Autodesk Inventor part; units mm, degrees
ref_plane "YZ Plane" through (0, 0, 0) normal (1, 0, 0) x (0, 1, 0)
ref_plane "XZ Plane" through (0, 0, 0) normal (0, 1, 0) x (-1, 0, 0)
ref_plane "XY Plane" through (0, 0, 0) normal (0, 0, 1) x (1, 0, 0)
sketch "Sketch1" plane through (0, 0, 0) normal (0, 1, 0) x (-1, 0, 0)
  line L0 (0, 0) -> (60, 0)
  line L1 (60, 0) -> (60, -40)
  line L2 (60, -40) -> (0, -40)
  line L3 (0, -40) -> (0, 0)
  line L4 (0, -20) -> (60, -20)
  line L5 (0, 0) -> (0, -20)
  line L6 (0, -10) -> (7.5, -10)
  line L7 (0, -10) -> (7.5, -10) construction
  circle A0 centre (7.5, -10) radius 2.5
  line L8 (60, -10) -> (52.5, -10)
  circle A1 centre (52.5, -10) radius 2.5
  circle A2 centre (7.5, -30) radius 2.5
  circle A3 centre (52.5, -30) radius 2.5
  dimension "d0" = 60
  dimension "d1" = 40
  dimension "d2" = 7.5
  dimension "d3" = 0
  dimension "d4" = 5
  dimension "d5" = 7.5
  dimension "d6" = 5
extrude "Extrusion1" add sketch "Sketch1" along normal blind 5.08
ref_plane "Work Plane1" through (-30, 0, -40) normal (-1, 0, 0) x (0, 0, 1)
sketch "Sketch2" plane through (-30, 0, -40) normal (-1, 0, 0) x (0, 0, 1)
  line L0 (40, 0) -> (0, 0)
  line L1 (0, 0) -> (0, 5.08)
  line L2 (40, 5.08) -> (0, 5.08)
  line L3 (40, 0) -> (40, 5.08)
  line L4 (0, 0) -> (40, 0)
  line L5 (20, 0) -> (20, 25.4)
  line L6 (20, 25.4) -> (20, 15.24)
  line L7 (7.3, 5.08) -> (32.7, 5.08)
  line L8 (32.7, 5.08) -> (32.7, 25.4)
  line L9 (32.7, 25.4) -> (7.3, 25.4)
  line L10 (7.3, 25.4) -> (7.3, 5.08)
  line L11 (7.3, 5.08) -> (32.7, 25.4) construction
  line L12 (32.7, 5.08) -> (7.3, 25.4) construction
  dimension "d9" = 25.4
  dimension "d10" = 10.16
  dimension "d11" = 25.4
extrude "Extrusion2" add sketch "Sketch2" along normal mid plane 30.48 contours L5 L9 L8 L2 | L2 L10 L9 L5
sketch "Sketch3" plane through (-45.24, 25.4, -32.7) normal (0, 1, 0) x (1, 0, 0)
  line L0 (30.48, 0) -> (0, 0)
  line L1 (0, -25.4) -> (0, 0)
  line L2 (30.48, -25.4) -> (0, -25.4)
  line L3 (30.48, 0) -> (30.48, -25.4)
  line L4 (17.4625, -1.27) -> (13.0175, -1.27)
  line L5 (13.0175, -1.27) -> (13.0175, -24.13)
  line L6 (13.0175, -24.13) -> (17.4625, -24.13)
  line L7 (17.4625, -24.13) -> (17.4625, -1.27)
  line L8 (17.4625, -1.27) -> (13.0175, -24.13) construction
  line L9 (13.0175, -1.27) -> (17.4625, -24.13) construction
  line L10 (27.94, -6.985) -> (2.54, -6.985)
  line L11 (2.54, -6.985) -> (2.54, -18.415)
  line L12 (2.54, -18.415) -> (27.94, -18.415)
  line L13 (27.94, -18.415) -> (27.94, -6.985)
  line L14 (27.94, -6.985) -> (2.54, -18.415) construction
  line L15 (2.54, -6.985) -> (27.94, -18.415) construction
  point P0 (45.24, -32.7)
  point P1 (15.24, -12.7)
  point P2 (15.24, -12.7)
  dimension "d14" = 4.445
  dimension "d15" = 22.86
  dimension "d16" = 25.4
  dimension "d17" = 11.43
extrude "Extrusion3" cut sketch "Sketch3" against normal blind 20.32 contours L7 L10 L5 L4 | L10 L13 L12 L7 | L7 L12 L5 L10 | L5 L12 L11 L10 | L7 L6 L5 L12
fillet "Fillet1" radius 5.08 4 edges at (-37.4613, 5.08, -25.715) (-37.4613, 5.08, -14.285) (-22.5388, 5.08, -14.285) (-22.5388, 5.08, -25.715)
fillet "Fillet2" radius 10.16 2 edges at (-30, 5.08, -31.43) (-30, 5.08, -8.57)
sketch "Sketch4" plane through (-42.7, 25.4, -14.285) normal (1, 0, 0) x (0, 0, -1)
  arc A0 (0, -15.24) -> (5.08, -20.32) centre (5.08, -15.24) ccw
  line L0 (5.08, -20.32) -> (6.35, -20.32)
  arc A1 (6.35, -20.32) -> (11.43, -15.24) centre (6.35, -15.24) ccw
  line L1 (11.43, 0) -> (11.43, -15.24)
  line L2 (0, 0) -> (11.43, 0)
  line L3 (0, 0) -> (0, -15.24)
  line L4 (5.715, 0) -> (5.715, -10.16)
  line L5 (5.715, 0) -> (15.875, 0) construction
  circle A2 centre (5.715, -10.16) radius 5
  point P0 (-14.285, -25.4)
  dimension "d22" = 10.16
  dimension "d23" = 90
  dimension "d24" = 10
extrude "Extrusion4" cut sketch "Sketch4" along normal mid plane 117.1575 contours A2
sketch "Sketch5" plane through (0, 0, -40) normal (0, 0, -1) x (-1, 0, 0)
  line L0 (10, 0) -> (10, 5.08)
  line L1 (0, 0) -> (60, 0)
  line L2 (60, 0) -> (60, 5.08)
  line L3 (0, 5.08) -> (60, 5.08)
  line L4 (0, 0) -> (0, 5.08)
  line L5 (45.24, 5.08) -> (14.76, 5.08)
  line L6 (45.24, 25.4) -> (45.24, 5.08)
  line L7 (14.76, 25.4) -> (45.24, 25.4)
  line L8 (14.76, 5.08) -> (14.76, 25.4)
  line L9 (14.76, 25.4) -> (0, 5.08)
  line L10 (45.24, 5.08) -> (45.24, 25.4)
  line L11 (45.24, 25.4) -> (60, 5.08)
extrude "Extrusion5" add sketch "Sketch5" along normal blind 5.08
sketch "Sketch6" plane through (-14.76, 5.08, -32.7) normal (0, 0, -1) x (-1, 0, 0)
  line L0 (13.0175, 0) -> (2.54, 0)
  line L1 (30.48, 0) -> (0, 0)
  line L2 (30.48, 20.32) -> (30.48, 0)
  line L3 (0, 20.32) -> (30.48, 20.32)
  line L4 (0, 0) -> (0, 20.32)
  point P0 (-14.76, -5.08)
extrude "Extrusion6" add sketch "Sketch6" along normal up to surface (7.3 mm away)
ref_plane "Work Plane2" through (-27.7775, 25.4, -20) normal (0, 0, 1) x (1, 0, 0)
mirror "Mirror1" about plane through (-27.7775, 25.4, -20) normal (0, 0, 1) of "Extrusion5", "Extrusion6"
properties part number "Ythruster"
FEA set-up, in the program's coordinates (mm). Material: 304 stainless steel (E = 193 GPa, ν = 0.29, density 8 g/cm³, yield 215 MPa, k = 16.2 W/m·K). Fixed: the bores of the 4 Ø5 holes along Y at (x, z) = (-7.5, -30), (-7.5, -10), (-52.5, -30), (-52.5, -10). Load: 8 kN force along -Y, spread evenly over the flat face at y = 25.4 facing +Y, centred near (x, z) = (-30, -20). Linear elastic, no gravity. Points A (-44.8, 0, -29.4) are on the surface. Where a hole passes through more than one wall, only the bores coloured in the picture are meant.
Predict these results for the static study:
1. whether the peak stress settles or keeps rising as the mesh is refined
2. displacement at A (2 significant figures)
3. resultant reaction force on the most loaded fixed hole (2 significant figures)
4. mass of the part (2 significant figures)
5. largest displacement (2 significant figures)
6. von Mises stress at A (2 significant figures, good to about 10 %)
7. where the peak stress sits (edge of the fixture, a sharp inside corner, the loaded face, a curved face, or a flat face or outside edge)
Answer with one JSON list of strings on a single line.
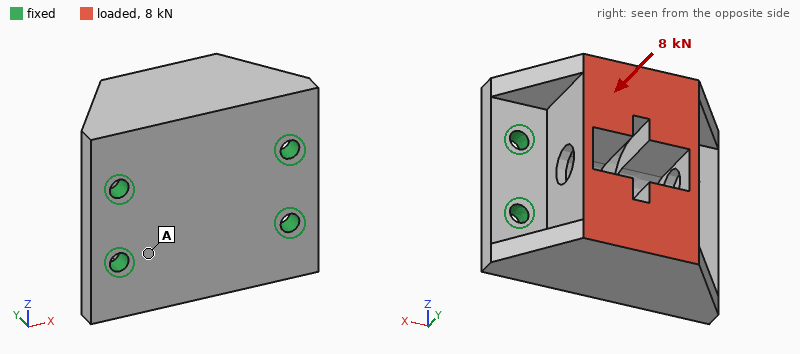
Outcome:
["keeps rising", "4.3 µm", "2.1 kN", "340 g", "8.1 µm", "23 MPa", "edge of the fixture"]
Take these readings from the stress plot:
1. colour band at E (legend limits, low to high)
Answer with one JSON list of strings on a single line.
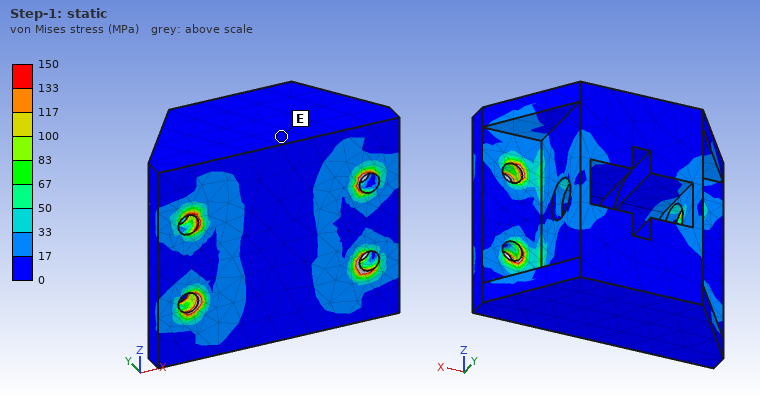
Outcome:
["0 to 17 MPa"]
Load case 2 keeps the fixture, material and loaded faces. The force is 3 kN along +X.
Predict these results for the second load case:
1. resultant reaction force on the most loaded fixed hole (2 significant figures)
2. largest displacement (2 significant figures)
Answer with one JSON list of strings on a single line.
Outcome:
["1.1 kN", "5.9 µm"]
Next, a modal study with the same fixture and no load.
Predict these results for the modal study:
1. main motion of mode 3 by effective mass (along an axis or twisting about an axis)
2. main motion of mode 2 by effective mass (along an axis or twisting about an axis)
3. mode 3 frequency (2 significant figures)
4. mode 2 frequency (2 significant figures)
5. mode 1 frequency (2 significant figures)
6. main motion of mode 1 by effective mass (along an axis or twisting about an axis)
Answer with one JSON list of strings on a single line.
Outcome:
["along X", "along Y", "12 kHz", "10 kHz", "6100 Hz", "along Z"]
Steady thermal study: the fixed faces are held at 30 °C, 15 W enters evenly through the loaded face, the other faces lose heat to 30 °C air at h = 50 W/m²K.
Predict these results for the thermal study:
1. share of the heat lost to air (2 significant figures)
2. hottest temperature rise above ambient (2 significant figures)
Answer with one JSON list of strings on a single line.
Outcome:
["46 %", "25 K"]
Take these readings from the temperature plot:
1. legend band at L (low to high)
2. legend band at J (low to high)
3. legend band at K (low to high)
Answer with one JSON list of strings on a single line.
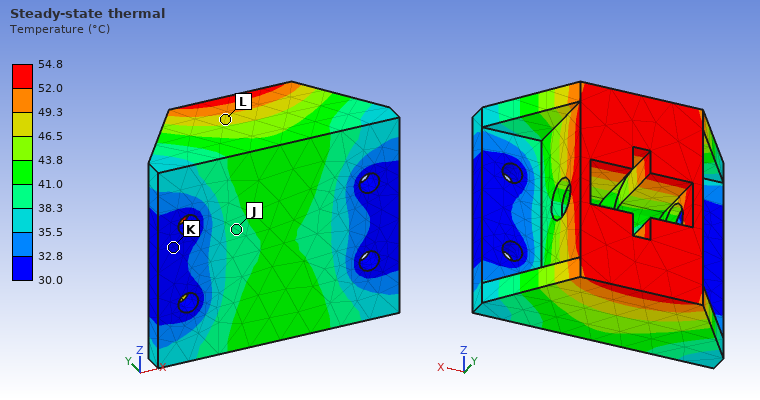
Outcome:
["46.5 to 49.3 °C", "38.3 to 41.0 °C", "30.0 to 32.8 °C"]
